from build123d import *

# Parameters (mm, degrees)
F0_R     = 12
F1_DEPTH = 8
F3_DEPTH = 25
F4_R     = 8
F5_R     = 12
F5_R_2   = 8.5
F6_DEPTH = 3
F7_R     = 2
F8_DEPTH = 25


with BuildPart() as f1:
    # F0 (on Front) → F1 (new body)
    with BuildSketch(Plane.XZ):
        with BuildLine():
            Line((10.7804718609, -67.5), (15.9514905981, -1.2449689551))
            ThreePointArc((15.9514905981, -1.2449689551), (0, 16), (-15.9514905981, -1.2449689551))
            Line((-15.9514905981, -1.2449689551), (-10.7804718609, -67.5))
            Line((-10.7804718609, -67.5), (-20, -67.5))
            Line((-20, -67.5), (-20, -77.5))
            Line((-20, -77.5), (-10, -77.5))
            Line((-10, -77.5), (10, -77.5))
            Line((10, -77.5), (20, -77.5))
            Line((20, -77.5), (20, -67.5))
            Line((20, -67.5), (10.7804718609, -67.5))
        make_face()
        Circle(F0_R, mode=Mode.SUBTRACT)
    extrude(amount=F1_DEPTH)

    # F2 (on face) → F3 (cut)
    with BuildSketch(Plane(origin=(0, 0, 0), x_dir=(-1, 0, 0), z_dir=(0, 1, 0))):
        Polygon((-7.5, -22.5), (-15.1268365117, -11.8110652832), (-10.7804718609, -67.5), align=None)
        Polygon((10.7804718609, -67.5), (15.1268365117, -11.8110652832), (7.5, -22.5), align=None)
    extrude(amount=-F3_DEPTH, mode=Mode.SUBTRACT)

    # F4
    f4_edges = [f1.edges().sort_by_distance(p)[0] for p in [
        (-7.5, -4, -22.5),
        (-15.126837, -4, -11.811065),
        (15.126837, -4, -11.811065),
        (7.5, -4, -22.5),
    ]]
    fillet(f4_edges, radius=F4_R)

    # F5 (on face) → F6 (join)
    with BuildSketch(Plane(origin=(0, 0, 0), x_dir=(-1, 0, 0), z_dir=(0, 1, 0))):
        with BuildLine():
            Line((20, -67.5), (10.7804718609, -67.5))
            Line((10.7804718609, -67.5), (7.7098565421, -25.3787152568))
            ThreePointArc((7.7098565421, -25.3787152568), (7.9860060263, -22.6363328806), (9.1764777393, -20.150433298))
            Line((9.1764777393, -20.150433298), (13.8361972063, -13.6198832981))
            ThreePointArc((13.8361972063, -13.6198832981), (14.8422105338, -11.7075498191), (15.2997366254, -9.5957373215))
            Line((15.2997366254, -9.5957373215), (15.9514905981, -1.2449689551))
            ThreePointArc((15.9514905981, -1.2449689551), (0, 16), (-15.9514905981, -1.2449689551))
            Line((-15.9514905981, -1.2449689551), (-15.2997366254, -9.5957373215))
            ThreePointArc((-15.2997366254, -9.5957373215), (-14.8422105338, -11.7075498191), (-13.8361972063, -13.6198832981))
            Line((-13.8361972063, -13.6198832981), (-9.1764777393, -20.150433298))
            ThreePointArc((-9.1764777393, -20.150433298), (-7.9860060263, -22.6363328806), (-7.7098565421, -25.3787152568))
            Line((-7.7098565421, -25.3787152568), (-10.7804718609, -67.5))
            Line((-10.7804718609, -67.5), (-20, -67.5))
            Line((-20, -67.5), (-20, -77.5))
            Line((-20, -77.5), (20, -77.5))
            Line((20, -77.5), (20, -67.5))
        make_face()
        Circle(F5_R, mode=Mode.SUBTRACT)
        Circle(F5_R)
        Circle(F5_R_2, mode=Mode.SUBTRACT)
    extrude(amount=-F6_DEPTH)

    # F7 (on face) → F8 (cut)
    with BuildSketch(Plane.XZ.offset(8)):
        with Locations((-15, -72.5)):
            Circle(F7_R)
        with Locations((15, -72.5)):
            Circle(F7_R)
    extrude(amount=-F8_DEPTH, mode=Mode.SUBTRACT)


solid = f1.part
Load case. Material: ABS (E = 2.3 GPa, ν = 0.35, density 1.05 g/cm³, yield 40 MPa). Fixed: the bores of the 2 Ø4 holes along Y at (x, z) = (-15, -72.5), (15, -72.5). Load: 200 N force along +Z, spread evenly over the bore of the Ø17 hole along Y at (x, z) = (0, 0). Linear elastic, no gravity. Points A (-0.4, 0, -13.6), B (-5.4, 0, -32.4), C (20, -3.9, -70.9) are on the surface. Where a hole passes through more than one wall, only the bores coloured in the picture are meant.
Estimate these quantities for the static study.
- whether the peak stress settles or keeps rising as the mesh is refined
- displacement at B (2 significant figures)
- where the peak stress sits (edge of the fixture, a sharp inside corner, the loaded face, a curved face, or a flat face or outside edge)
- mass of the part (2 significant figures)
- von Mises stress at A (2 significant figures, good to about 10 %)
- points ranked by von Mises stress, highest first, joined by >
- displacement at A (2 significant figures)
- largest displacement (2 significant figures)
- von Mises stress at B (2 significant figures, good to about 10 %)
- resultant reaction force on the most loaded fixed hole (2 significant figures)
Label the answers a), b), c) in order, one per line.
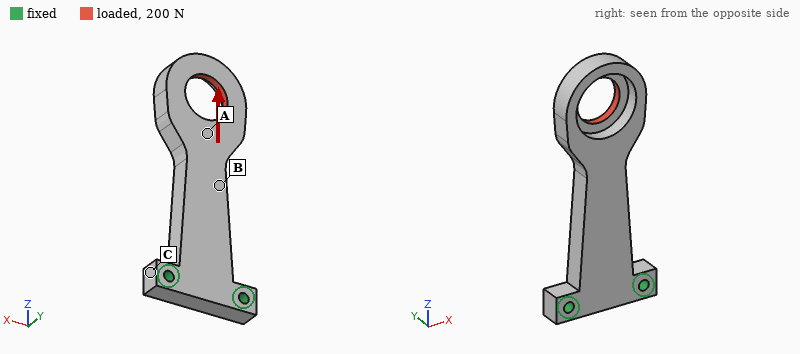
a) keeps rising
b) 0.28 mm
c) edge of the fixture
d) 15 g
e) 2.4 MPa
f) B > A > C
g) 0.56 mm
h) 1.2 mm
i) 4.4 MPa
j) 110 N
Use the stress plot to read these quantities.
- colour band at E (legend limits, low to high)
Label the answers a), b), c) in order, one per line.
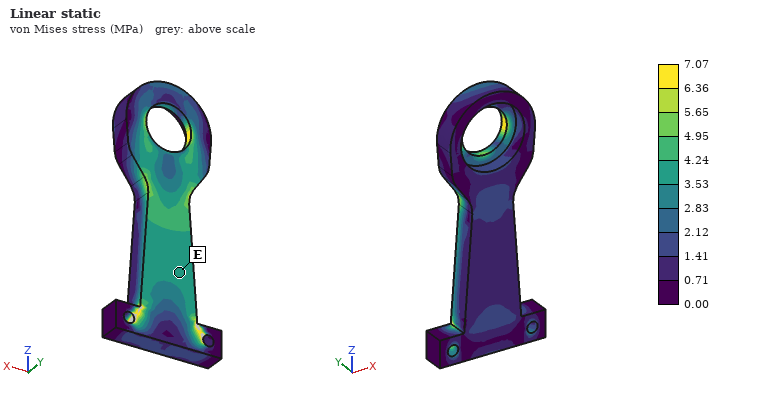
a) 3.53 to 4.24 MPa
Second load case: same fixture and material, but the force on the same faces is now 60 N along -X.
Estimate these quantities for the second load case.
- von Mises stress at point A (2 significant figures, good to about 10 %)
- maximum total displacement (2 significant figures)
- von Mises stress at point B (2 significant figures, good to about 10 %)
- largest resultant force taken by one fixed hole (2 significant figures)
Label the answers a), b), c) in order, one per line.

a) 3.0 MPa
b) 1.1 mm
c) 3.8 MPa
d) 170 N
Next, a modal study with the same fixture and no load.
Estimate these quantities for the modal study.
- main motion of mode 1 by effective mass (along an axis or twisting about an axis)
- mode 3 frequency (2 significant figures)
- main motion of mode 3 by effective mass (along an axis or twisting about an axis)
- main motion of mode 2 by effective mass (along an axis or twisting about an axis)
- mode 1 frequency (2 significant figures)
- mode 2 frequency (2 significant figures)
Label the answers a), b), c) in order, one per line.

a) along Y
b) 1200 Hz
c) twisting about Z
d) along X
e) 240 Hz
f) 620 Hz
